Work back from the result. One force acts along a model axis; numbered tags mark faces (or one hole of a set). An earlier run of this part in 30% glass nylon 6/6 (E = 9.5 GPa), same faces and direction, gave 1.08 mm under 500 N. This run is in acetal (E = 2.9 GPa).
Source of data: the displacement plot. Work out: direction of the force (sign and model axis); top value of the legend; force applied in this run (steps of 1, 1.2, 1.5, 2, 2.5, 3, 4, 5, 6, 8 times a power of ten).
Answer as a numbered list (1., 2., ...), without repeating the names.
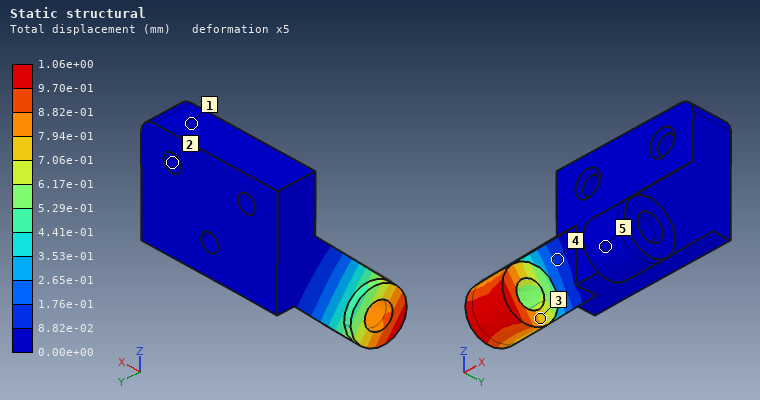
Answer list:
1. -X
2. 1.06e+00 mm
3. 150 N
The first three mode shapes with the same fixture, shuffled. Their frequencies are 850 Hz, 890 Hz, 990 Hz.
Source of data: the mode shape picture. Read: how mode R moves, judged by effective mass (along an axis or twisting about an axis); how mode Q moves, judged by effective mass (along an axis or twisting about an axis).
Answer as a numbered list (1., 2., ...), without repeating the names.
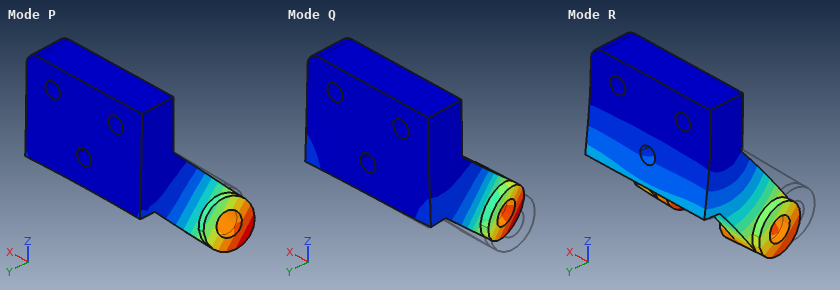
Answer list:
1. along Y
2. along X
